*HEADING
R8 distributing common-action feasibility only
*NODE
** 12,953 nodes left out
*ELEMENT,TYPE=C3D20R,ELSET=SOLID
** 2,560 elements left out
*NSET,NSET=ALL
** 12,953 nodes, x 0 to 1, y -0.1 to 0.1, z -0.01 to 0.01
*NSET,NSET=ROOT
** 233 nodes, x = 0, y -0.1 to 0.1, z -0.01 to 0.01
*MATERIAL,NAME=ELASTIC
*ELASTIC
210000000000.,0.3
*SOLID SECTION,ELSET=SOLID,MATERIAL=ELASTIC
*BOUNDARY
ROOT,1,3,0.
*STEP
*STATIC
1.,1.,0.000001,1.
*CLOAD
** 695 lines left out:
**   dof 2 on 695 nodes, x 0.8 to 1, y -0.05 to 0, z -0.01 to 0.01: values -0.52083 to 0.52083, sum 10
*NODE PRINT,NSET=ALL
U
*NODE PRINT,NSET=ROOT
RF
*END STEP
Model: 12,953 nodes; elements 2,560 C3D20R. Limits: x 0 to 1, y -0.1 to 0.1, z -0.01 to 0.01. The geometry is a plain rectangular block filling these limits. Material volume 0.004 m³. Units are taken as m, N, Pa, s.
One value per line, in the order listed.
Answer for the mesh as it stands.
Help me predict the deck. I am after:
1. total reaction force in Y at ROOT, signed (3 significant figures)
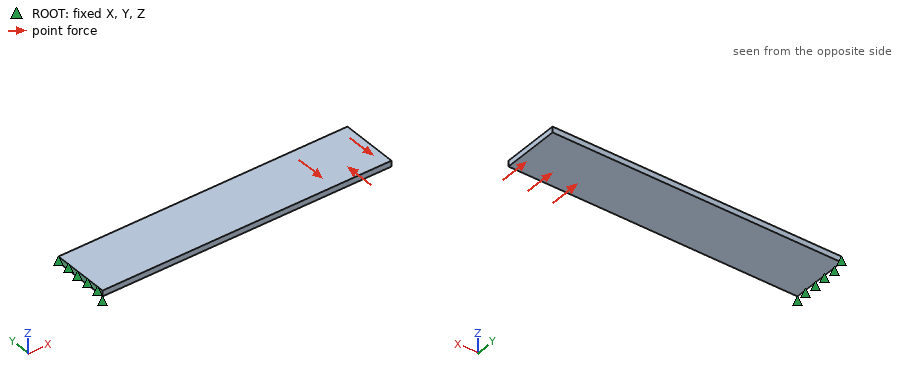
-10.0 N
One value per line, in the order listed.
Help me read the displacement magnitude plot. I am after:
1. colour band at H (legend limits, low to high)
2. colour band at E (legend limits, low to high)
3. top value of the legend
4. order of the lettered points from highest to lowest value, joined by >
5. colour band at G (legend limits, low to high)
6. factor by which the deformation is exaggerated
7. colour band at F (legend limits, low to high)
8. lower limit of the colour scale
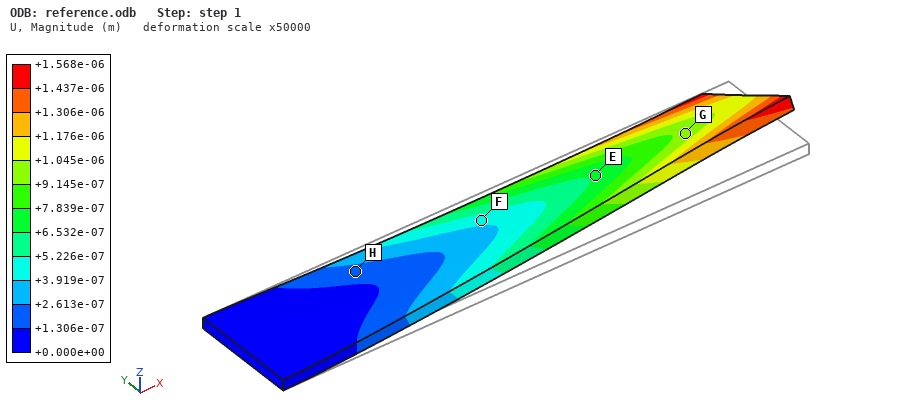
+1.306e-07 to +2.613e-07 m
+6.532e-07 to +7.839e-07 m
+1.568e-06 m
G > E > F > H
+9.145e-07 to +1.045e-06 m
50000
+3.919e-07 to +5.226e-07 m
+0.000e+00 m
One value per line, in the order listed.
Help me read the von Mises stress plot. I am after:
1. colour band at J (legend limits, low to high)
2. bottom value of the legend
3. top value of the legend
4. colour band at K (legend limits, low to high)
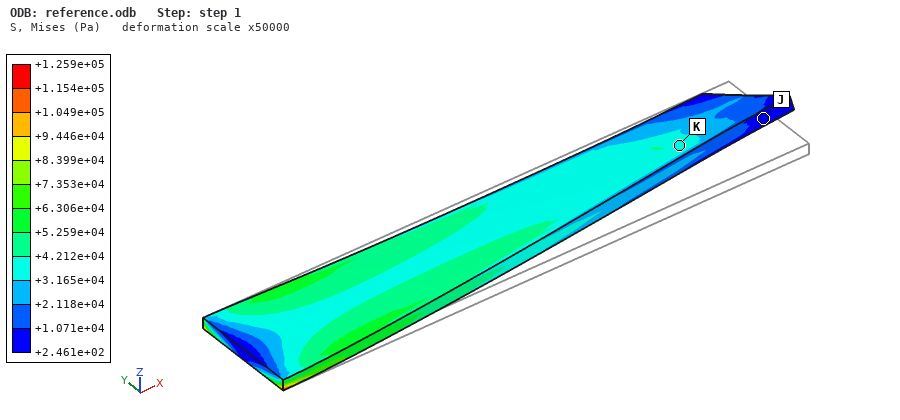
+2.461e+02 to +1.071e+04 Pa
+2.461e+02 Pa
+1.259e+05 Pa
+3.165e+04 to +4.212e+04 Pa
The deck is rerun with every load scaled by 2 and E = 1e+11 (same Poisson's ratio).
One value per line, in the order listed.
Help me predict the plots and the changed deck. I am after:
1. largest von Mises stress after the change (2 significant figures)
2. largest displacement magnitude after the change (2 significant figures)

2.5e+05 Pa
6.6e-06 m
